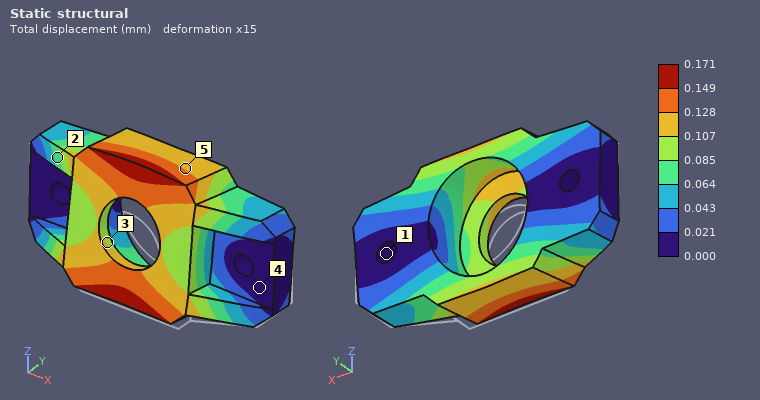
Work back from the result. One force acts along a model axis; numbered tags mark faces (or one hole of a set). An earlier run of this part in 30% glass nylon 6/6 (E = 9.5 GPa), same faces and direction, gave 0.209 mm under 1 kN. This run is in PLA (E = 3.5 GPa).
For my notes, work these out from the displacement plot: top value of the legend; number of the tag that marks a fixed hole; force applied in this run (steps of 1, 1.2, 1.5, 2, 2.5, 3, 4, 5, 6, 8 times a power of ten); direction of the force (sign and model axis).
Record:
0.171 mm
1
300 N
+Z
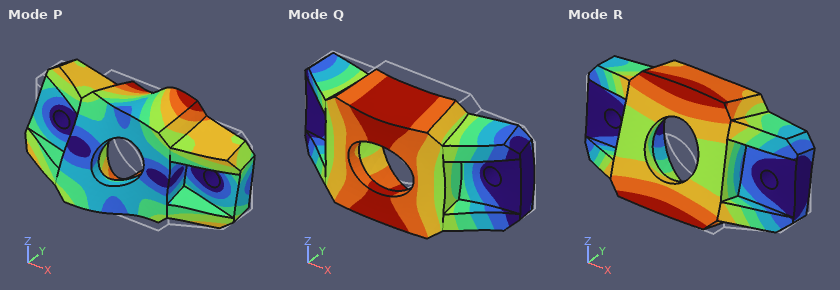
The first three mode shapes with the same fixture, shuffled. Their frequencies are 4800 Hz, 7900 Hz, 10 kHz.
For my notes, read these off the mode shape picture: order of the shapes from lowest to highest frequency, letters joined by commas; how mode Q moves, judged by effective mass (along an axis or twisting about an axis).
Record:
R, Q, P
along Y
